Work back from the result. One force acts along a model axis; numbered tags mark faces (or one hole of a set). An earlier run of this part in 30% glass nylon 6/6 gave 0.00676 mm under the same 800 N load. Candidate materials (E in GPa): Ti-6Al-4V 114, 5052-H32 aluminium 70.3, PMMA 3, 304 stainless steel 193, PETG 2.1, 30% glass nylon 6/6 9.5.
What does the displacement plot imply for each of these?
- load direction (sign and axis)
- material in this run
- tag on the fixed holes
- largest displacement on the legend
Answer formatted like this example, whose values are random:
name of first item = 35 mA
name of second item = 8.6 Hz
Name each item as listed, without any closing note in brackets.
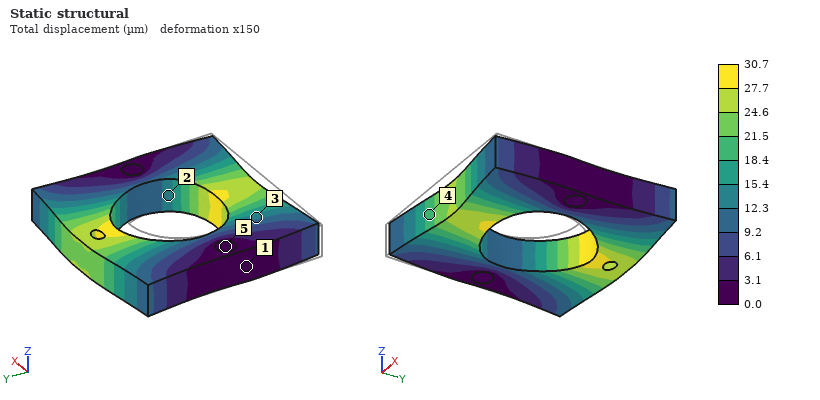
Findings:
load direction = +Y
material in this run = PETG
tag on the fixed holes = 5
largest displacement on the legend = 30.7 µm
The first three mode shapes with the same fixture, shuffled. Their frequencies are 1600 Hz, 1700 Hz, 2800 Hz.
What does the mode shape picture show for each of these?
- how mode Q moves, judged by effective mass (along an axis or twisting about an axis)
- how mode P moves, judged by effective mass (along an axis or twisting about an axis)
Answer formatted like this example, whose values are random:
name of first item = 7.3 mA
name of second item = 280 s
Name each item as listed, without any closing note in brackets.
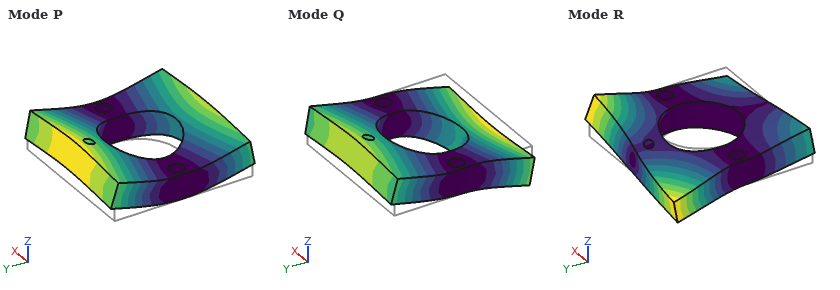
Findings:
how mode Q moves, judged by effective mass = twisting about X
how mode P moves, judged by effective mass = along Z
